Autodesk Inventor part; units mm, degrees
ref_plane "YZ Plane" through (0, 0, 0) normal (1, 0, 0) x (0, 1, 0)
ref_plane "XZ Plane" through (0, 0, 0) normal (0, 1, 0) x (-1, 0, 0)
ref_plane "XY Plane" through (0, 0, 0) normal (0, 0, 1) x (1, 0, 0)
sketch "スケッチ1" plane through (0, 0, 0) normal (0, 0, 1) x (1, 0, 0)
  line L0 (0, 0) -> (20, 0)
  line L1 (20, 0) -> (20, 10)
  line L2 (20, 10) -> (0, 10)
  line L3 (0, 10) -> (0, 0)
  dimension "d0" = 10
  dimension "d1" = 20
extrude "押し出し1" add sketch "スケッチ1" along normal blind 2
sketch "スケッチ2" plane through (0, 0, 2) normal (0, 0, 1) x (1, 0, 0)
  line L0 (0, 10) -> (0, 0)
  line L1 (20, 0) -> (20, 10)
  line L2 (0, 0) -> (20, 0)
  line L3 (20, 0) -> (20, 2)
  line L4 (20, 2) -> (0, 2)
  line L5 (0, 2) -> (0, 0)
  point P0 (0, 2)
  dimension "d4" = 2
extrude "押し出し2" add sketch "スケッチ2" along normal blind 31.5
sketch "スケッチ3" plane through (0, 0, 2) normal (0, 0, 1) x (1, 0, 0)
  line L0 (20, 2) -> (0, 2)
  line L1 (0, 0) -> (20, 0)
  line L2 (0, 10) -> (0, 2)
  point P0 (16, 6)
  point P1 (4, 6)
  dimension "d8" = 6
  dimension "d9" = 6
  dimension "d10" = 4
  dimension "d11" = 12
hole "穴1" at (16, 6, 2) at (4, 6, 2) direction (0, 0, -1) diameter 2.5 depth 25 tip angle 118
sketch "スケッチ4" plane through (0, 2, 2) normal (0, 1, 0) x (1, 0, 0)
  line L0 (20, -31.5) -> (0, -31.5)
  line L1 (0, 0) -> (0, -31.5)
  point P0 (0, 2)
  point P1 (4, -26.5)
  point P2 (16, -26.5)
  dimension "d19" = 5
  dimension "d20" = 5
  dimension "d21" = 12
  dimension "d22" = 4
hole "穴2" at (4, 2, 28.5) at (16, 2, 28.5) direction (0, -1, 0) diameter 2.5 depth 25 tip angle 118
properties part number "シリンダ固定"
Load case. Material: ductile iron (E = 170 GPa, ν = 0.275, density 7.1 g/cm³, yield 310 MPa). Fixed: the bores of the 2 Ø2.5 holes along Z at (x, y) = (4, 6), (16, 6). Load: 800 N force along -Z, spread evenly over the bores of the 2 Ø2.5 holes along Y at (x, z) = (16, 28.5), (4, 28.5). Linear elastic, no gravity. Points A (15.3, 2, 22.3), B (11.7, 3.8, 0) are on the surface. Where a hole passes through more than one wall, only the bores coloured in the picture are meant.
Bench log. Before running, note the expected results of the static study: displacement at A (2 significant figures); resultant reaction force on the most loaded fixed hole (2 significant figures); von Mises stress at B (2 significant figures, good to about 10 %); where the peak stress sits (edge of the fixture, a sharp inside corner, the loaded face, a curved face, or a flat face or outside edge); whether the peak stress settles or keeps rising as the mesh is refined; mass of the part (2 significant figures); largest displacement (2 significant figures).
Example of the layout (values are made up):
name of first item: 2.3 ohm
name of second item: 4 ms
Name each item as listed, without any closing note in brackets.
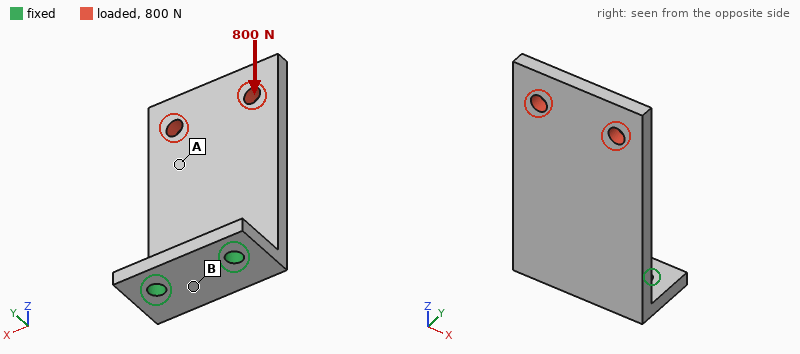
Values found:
displacement at A: 0.085 mm
resultant reaction force on the most loaded fixed hole: 400 N
von Mises stress at B: 97 MPa
where the peak stress sits: edge of the fixture
whether the peak stress settles or keeps rising as the mesh is refined: keeps rising
mass of the part: 12 g
largest displacement: 0.13 mm
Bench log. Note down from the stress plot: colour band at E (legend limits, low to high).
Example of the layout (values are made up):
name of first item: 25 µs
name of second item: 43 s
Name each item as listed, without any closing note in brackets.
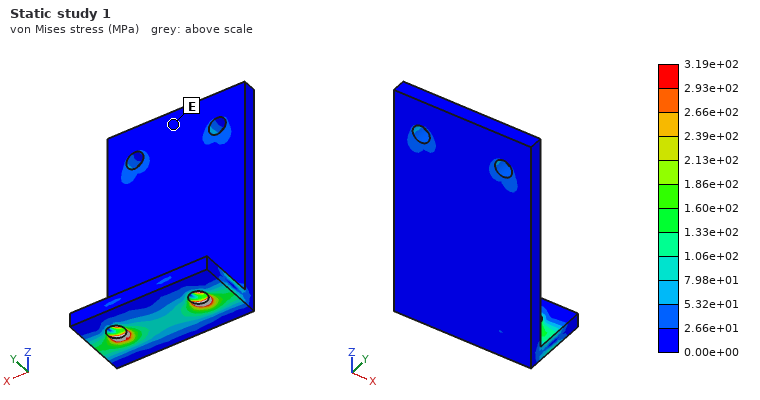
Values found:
colour band at E: 0.00e+00 to 2.66e+01 MPa
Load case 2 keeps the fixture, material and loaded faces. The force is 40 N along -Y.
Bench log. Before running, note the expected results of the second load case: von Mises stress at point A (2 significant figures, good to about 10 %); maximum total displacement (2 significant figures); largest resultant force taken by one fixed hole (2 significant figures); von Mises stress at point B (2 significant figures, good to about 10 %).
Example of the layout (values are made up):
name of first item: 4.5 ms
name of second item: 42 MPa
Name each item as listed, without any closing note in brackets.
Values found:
von Mises stress at point A: 19 MPa
maximum total displacement: 0.21 mm
largest resultant force taken by one fixed hole: 24 N
von Mises stress at point B: 59 MPa
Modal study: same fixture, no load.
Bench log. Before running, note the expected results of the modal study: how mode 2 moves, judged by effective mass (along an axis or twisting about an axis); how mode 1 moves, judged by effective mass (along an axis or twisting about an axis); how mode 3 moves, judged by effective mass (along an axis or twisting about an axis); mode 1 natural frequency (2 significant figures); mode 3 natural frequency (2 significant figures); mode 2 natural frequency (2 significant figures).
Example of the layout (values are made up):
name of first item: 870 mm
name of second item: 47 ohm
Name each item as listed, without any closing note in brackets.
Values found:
how mode 2 moves, judged by effective mass: along X
how mode 1 moves, judged by effective mass: along Y
how mode 3 moves, judged by effective mass: along X
mode 1 natural frequency: 1300 Hz
mode 3 natural frequency: 5800 Hz
mode 2 natural frequency: 4500 Hz
